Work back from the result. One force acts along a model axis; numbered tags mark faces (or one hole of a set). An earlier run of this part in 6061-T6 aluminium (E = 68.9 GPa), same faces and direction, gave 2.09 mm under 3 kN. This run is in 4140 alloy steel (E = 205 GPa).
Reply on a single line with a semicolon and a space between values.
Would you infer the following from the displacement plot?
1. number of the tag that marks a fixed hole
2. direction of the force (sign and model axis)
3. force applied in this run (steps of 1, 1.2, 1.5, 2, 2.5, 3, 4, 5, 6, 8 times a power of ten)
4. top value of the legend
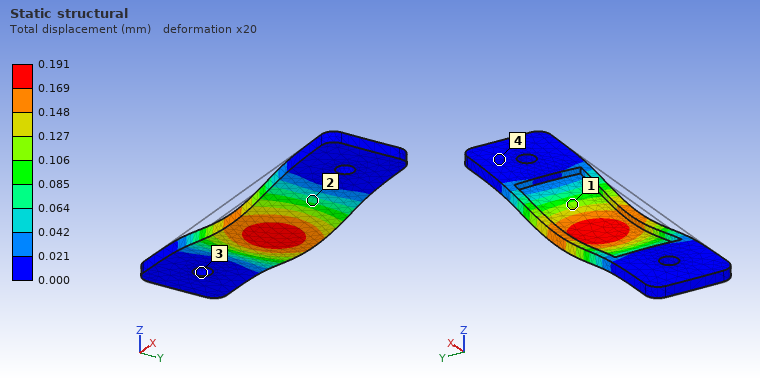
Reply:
3; -Z; 800 N; 0.191 mm
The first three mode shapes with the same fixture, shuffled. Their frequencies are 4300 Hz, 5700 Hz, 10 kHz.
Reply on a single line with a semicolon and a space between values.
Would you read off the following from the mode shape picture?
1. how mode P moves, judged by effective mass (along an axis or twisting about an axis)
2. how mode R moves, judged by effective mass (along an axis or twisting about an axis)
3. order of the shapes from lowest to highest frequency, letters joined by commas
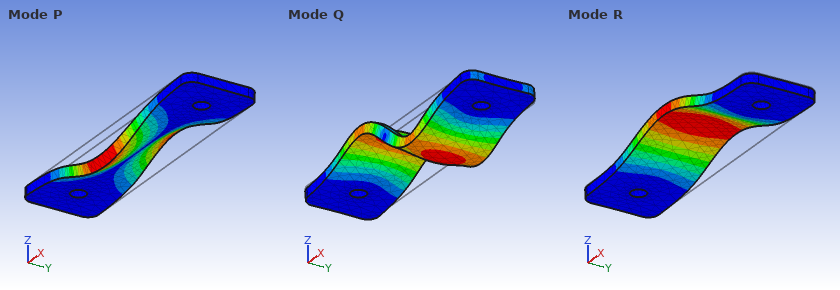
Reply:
twisting about X; along Z; R, P, Q
